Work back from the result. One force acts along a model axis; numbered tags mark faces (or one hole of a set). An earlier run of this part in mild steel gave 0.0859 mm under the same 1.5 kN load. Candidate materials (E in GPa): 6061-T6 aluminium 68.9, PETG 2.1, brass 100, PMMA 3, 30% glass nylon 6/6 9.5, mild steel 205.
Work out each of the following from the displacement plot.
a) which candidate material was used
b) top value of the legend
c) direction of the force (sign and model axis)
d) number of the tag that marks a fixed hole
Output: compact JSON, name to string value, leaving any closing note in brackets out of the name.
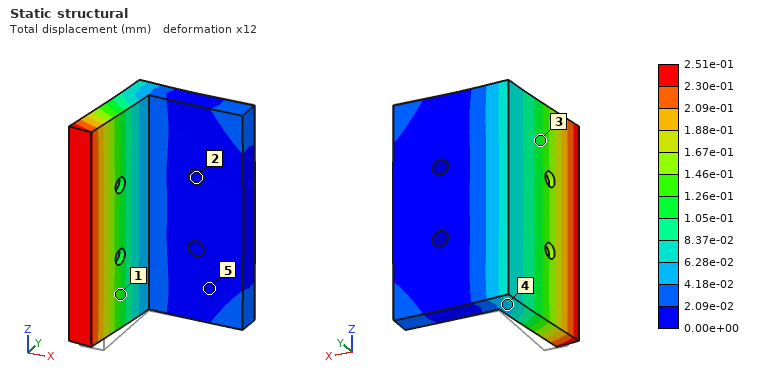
{"which candidate material was used": "6061-T6 aluminium", "top value of the legend": "2.51e-01 mm", "direction of the force": "-X", "number of the tag that marks a fixed hole": "2"}
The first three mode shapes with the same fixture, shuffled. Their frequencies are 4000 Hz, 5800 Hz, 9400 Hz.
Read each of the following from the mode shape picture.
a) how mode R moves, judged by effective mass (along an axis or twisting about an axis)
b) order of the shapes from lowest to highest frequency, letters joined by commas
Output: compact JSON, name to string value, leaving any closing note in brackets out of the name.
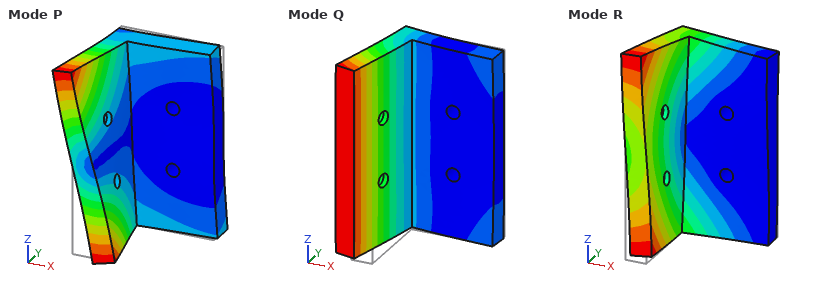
{"how mode R moves, judged by effective mass": "along Z", "order of the shapes from lowest to highest frequency, letters joined by commas": "Q, R, P"}
